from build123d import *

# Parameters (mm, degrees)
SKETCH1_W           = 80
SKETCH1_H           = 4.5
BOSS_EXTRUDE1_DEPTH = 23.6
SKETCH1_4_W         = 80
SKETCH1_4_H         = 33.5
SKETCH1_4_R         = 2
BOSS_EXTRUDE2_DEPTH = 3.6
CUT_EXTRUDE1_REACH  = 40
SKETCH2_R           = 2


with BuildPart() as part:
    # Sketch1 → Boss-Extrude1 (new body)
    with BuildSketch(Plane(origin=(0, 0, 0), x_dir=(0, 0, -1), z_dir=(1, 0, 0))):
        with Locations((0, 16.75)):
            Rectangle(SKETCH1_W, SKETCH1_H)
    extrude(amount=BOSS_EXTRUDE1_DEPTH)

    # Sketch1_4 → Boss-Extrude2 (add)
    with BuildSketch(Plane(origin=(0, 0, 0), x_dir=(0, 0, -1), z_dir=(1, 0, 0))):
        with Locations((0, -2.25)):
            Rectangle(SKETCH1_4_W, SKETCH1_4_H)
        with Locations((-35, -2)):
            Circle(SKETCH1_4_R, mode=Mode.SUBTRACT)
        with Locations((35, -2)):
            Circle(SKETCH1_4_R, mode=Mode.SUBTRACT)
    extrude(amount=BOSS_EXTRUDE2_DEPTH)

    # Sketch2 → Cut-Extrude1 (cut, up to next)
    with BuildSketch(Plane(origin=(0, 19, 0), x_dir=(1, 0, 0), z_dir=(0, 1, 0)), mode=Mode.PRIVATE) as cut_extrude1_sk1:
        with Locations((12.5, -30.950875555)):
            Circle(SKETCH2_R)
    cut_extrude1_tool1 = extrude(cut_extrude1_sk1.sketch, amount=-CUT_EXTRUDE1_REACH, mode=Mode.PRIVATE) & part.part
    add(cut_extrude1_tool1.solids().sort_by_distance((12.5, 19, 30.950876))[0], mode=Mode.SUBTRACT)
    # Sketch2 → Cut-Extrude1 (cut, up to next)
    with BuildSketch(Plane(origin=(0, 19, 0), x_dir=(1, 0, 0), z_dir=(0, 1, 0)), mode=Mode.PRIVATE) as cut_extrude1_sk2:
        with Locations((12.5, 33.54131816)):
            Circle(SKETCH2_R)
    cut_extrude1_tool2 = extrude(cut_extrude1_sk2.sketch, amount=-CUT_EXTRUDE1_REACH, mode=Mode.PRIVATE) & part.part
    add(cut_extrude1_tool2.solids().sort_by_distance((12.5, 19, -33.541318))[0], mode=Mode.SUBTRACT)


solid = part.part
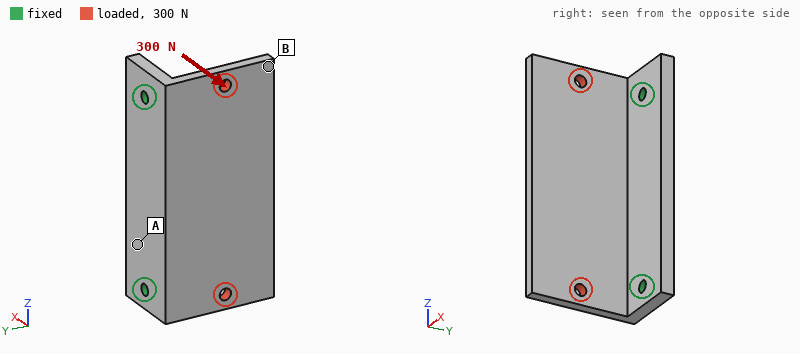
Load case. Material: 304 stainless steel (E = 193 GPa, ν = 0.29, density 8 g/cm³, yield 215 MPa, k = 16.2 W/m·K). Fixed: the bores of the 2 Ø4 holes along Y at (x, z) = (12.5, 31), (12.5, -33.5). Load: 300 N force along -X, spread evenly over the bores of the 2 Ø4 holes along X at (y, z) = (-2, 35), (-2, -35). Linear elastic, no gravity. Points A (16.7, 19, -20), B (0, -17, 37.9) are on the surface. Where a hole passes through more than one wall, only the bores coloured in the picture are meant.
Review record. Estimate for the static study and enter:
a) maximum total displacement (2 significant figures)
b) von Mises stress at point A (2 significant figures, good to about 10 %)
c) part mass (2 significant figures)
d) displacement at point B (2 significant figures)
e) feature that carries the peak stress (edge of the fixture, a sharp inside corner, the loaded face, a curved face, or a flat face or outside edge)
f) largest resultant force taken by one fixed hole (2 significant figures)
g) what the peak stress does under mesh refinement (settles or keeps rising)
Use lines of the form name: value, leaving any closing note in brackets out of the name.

maximum total displacement: 58 µm
von Mises stress at point A: 9.7 MPa
part mass: 140 g
displacement at point B: 53 µm
feature that carries the peak stress: edge of the fixture
largest resultant force taken by one fixed hole: 160 N
what the peak stress does under mesh refinement: keeps rising
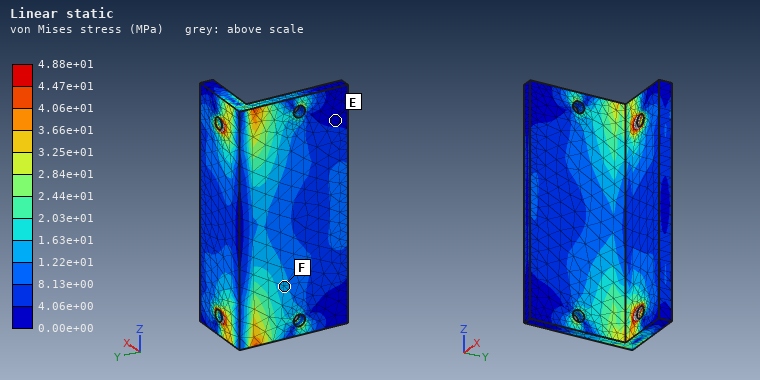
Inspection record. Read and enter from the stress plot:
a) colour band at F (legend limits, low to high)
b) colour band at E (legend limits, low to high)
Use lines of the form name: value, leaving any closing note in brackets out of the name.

colour band at F: 1.22e+01 to 1.63e+01 MPa
colour band at E: 0.00e+00 to 4.06e+00 MPa
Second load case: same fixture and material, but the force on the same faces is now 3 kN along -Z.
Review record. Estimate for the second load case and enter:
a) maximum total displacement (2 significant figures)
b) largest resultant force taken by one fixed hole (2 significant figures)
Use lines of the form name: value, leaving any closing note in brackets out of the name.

maximum total displacement: 36 µm
largest resultant force taken by one fixed hole: 1.8 kN
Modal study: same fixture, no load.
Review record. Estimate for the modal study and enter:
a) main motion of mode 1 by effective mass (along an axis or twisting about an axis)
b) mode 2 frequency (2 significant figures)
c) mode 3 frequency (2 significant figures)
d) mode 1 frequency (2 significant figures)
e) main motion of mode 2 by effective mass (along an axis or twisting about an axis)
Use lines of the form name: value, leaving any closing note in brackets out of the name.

main motion of mode 1 by effective mass: along X
mode 2 frequency: 2800 Hz
mode 3 frequency: 5300 Hz
mode 1 frequency: 1600 Hz
main motion of mode 2 by effective mass: twisting about Y
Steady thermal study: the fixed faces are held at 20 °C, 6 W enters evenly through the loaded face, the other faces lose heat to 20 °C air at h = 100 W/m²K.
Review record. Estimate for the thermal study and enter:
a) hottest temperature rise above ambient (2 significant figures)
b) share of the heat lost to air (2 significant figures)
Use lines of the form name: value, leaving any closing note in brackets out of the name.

hottest temperature rise above ambient: 29 K
share of the heat lost to air: 85 %
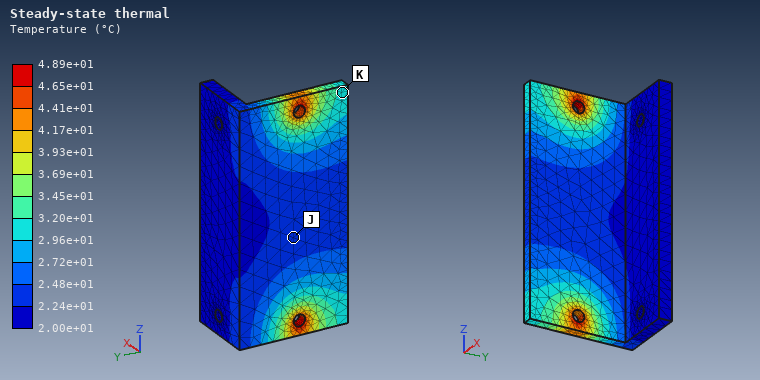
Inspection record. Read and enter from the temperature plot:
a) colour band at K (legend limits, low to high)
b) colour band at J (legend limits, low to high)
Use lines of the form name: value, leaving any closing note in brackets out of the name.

colour band at K: 2.96e+01 to 3.20e+01 °C
colour band at J: 2.24e+01 to 2.48e+01 °C
